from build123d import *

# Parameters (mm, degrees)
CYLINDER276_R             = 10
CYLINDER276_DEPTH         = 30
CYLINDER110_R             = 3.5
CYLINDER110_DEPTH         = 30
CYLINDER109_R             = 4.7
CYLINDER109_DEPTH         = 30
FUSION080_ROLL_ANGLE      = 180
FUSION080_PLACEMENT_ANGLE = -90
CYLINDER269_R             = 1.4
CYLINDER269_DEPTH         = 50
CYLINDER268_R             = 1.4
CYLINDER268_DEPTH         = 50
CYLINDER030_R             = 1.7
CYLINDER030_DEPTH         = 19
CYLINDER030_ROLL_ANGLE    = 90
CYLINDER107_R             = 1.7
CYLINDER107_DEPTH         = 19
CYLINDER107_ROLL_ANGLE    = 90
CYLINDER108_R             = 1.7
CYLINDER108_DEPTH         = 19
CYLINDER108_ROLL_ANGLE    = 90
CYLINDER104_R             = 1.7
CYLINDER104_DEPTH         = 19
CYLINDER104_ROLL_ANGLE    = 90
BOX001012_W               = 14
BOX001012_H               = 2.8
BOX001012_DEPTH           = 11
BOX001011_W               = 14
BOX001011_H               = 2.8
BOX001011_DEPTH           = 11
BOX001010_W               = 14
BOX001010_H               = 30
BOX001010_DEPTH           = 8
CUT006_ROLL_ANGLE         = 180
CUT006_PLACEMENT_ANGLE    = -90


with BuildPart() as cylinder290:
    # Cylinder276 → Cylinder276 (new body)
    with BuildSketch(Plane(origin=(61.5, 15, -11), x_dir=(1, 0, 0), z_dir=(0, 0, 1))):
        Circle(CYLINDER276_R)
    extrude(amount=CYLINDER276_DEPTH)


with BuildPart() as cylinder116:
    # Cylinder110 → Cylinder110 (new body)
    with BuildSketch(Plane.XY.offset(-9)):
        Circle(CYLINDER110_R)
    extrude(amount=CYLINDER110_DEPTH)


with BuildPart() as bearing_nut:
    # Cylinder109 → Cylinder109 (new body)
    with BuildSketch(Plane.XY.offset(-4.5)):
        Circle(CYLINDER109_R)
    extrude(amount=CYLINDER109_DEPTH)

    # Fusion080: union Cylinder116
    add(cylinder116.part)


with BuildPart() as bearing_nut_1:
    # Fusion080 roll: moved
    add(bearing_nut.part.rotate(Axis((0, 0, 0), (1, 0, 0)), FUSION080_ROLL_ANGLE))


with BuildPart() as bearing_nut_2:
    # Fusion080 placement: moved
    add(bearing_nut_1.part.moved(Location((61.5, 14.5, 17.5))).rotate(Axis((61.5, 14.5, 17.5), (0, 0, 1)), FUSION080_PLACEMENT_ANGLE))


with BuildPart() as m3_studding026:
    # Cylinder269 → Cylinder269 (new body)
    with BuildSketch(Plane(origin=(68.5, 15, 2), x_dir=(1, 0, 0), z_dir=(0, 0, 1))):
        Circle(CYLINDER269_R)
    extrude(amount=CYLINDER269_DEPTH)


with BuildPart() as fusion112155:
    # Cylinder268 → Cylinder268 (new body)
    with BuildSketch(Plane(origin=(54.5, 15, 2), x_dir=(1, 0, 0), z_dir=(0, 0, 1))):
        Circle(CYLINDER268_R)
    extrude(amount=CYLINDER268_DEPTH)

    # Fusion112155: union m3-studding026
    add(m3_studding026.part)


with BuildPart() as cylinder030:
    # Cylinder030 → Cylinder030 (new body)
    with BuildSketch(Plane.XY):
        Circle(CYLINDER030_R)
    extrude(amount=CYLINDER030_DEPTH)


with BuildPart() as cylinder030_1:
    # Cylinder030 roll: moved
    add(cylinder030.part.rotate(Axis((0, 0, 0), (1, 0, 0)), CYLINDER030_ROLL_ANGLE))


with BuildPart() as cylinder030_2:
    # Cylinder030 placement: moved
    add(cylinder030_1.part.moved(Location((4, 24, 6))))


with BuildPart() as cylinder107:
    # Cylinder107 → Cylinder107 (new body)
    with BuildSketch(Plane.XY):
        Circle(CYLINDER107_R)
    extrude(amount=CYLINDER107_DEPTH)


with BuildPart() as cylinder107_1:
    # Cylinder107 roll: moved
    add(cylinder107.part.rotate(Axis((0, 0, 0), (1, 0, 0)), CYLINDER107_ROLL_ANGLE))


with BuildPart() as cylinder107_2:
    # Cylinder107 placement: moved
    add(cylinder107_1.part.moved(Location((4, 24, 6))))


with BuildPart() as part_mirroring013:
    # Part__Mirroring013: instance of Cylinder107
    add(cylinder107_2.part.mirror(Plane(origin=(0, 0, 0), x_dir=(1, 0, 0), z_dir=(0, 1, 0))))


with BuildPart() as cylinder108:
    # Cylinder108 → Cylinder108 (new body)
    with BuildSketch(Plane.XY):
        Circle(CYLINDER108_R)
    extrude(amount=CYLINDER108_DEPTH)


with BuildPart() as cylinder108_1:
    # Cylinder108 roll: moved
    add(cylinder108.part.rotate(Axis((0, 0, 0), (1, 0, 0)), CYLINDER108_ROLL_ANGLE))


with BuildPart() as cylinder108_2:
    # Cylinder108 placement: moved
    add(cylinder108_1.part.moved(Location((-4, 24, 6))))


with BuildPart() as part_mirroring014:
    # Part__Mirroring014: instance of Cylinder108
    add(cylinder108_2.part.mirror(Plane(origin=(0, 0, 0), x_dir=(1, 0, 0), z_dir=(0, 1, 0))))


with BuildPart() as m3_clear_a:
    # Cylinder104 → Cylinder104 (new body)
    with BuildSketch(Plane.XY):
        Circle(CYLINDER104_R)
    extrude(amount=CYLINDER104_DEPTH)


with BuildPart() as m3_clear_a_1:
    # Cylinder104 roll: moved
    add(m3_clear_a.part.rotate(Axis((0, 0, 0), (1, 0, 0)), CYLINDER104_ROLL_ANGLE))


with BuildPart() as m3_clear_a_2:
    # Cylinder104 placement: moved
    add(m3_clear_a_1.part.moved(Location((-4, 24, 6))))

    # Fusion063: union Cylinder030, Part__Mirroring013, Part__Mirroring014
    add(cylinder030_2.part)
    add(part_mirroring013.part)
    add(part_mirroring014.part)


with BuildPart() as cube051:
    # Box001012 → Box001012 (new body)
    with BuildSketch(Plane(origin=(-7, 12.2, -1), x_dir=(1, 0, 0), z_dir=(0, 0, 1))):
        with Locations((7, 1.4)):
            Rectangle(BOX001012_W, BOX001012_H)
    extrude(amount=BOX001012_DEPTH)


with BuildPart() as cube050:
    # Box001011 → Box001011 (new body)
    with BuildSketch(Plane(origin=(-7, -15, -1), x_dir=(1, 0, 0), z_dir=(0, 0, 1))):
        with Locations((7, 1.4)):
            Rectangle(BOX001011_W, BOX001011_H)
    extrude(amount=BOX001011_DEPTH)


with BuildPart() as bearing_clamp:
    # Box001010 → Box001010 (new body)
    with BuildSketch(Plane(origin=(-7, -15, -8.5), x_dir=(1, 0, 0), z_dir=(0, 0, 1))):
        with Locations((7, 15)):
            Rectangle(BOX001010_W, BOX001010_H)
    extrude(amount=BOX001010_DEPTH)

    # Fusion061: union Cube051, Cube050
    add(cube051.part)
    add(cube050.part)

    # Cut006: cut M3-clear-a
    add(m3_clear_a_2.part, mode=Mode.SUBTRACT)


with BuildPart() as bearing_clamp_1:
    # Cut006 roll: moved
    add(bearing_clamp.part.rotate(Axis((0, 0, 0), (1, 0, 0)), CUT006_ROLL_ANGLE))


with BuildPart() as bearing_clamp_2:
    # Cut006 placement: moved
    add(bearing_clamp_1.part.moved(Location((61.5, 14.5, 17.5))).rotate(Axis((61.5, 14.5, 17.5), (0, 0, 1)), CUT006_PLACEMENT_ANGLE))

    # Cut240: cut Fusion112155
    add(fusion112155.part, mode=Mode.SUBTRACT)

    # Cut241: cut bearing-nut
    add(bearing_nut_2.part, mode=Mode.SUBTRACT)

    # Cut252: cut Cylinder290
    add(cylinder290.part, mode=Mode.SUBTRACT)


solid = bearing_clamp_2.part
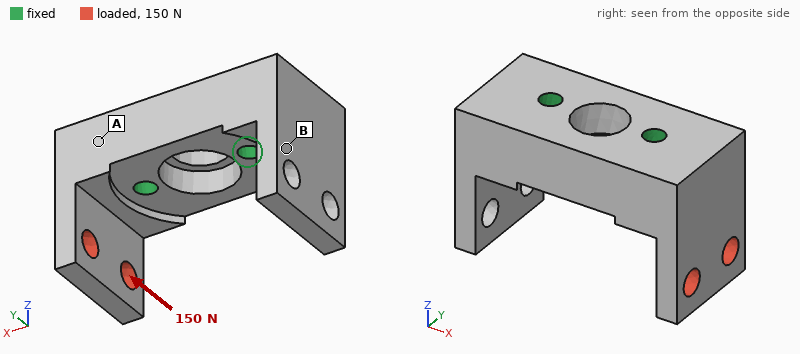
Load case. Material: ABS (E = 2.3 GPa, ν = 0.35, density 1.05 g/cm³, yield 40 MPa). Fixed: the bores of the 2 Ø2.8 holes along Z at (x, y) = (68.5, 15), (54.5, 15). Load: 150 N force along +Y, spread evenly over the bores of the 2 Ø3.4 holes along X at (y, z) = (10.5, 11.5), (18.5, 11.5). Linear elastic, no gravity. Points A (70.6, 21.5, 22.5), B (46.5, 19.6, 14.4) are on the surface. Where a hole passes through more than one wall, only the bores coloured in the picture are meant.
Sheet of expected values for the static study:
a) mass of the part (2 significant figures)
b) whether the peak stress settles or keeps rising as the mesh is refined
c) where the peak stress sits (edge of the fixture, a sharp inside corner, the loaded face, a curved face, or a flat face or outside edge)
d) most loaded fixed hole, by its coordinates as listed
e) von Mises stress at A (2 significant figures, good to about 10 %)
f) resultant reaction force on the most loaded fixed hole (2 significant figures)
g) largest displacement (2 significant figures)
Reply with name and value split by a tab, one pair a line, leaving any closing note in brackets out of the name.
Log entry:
mass of the part	3.5 g
whether the peak stress settles or keeps rising as the mesh is refined	keeps rising
where the peak stress sits	edge of the fixture
most loaded fixed hole, by its coordinates as listed	(68.5, 15)
von Mises stress at A	10 MPa
resultant reaction force on the most loaded fixed hole	180 N
largest displacement	0.31 mm
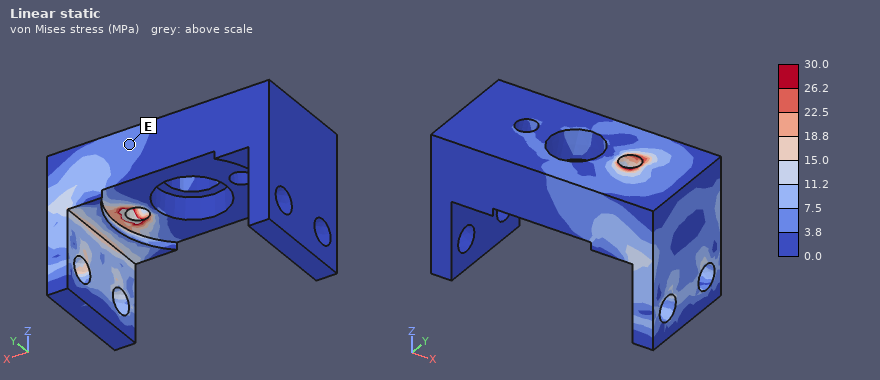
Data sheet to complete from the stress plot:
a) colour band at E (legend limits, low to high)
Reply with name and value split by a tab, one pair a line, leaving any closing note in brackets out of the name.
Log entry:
colour band at E	3.8 to 7.5 MPa
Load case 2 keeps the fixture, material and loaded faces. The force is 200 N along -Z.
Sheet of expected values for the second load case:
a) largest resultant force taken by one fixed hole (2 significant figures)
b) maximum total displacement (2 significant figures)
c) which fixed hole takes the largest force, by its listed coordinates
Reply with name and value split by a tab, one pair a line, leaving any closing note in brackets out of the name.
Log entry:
largest resultant force taken by one fixed hole	220 N
maximum total displacement	0.15 mm
which fixed hole takes the largest force, by its listed coordinates	(68.5, 15)
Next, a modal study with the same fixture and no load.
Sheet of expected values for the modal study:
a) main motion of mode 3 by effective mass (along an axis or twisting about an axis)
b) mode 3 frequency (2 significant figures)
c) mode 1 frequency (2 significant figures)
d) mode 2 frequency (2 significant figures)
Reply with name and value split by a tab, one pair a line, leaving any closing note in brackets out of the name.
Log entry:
main motion of mode 3 by effective mass	twisting about Z
mode 3 frequency	6600 Hz
mode 1 frequency	4400 Hz
mode 2 frequency	4400 Hz
